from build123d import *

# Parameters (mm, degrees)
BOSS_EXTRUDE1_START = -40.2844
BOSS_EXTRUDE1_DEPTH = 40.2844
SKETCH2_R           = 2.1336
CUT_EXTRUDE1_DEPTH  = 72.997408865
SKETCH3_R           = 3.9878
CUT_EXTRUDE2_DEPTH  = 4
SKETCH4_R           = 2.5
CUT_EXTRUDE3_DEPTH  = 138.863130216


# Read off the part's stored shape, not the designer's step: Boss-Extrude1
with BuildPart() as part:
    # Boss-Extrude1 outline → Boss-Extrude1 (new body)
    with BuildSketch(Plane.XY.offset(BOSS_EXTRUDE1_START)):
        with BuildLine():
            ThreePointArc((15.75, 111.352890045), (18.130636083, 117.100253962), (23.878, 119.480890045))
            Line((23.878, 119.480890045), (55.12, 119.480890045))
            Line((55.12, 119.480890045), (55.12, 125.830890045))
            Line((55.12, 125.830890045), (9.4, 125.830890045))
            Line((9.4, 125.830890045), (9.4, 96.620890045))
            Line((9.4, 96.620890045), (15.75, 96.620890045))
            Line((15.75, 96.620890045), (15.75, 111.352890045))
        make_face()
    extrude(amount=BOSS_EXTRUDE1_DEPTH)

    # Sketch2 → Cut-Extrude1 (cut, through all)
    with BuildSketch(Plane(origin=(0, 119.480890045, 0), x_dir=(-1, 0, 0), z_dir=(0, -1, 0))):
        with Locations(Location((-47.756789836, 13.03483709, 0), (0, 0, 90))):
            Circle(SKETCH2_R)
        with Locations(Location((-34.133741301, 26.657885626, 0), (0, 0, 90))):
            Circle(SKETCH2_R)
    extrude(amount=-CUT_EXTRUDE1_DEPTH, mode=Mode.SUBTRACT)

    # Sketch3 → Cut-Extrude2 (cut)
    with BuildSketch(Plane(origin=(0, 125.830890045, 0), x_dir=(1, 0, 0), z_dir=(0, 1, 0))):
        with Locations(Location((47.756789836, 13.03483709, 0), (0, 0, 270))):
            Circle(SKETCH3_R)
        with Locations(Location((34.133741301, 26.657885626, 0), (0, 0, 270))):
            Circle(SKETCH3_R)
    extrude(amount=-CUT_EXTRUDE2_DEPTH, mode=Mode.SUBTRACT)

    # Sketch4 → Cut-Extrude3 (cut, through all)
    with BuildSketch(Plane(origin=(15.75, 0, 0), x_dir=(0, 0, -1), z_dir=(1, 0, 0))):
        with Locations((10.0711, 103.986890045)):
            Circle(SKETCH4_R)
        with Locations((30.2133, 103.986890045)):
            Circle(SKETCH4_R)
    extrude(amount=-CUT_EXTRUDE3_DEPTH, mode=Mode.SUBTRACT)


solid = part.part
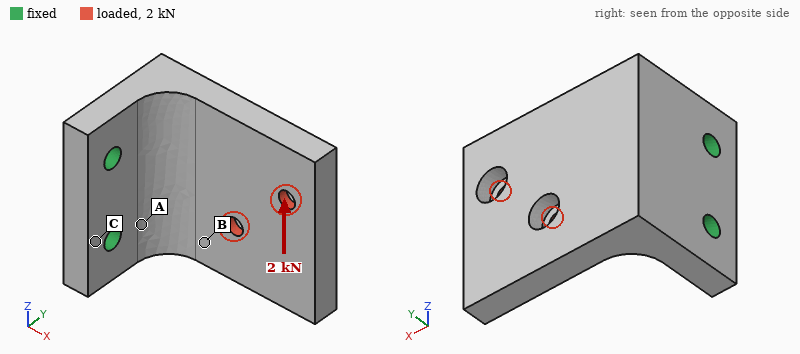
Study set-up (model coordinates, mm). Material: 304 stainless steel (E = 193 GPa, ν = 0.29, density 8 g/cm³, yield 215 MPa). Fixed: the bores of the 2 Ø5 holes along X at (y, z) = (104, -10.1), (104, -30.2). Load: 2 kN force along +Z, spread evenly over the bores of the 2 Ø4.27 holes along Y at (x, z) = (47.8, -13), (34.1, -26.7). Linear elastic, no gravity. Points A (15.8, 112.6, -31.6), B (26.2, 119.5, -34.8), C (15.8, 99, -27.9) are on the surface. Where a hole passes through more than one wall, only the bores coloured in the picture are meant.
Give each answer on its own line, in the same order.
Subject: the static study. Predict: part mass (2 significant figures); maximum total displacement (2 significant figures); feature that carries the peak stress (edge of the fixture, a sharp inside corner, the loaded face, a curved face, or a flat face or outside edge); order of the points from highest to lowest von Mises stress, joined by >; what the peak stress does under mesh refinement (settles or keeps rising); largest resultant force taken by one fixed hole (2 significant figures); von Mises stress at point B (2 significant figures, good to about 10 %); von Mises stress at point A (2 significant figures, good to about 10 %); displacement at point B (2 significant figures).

140 g
77 µm
edge of the fixture
A > B > C
keeps rising
2.7 kN
51 MPa
87 MPa
31 µm
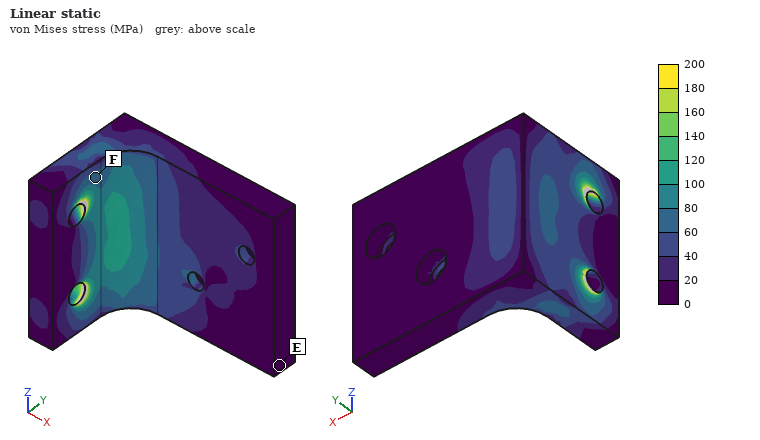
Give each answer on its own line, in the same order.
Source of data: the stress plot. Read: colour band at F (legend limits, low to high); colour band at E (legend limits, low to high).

60 to 80 MPa
0 to 20 MPa
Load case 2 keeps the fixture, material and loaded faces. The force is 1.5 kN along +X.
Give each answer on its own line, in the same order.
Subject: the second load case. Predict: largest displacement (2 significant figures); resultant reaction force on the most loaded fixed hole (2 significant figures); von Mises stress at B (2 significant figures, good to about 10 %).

45 µm
770 N
15 MPa
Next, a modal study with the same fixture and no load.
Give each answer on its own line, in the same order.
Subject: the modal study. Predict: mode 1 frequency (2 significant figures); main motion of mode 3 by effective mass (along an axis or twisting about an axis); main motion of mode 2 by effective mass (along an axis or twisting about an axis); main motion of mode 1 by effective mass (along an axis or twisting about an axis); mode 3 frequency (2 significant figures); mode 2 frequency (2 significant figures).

2000 Hz
along X
along Z
along Y
6700 Hz
3900 Hz
